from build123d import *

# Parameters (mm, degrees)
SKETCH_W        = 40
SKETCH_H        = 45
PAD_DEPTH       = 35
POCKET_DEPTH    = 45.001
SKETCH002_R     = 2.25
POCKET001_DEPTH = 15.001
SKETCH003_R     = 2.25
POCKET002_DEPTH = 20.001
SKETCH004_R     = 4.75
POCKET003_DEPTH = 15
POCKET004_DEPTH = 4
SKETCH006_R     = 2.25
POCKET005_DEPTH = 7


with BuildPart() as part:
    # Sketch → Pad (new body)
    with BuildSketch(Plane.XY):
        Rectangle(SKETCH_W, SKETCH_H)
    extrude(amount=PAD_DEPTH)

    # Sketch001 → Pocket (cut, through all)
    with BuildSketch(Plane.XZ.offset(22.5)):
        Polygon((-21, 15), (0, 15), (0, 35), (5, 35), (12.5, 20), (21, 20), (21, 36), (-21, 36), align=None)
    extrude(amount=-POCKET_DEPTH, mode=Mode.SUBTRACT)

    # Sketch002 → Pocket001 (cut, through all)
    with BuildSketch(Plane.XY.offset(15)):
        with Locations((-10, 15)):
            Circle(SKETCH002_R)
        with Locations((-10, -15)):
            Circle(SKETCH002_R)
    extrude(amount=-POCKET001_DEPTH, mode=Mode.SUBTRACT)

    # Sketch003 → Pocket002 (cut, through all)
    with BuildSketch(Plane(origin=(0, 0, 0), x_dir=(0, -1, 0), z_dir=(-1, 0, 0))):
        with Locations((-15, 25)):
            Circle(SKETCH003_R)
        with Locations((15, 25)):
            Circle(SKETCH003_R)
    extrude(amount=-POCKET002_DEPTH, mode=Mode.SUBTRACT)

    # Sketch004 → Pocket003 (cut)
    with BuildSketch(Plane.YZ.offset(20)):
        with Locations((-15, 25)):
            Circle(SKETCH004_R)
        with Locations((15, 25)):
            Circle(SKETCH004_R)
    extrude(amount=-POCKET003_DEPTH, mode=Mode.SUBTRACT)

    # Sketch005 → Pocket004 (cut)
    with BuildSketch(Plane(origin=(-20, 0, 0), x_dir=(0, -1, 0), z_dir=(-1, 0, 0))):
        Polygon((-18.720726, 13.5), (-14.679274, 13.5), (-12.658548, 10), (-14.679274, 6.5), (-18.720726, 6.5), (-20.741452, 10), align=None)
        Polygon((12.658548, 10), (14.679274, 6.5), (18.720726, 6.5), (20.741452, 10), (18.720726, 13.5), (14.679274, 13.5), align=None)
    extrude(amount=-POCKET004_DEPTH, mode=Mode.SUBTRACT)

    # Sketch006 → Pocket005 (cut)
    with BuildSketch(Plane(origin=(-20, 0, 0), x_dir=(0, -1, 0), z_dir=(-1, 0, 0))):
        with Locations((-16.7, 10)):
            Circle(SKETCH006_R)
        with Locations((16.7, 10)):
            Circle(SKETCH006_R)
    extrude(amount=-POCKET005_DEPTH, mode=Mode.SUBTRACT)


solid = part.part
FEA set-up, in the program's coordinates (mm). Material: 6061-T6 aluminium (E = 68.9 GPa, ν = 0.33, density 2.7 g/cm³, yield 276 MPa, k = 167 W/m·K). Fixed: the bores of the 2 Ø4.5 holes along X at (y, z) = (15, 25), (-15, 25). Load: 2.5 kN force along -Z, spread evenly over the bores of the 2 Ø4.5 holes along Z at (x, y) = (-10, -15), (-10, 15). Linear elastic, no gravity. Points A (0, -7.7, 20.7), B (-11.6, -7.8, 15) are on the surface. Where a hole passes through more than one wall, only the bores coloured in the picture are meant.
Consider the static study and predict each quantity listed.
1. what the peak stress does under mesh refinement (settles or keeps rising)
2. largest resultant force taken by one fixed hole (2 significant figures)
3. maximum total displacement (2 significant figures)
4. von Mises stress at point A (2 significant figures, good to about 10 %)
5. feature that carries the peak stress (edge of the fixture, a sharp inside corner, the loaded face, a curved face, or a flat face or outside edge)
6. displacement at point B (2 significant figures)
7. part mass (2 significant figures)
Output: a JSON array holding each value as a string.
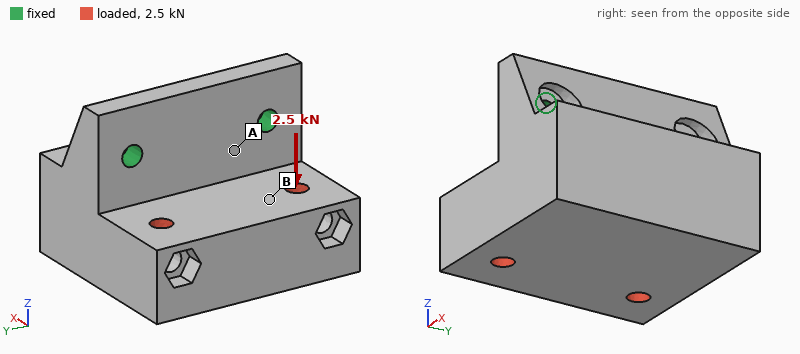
["keeps rising", "1.3 kN", "0.12 mm", "39 MPa", "edge of the fixture", "0.064 mm", "96 g"]
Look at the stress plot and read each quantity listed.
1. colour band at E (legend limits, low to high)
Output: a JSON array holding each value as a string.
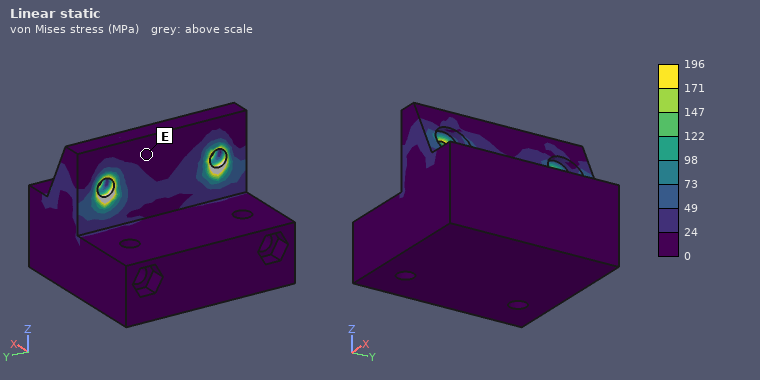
["0 to 24 MPa"]
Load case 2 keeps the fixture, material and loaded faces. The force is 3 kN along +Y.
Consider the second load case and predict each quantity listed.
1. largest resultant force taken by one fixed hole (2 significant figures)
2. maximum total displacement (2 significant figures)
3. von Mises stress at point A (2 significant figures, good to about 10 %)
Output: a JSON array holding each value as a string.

["2.5 kN", "33 µm", "38 MPa"]
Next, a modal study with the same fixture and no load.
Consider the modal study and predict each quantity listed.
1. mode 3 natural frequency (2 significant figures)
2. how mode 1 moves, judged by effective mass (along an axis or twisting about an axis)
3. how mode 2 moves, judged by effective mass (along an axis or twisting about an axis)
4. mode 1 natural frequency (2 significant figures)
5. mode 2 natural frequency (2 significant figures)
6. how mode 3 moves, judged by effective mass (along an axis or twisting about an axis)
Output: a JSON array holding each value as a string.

["12 kHz", "along X", "along Y", "2800 Hz", "8000 Hz", "along Y"]
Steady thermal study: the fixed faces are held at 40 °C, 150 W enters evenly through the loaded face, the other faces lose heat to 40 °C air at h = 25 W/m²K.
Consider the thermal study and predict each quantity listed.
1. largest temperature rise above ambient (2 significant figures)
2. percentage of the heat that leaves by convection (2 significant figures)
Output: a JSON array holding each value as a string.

["61 K", "5.1 %"]
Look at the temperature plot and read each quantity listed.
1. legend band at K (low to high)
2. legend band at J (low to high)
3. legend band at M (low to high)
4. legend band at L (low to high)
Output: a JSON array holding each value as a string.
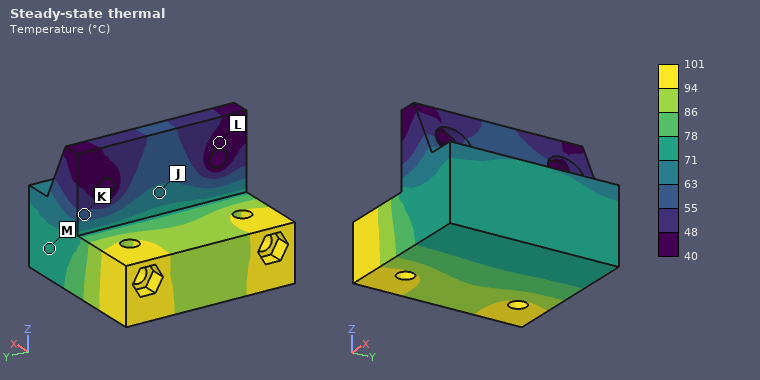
["55 to 63 °C", "63 to 71 °C", "71 to 78 °C", "40 to 48 °C"]
